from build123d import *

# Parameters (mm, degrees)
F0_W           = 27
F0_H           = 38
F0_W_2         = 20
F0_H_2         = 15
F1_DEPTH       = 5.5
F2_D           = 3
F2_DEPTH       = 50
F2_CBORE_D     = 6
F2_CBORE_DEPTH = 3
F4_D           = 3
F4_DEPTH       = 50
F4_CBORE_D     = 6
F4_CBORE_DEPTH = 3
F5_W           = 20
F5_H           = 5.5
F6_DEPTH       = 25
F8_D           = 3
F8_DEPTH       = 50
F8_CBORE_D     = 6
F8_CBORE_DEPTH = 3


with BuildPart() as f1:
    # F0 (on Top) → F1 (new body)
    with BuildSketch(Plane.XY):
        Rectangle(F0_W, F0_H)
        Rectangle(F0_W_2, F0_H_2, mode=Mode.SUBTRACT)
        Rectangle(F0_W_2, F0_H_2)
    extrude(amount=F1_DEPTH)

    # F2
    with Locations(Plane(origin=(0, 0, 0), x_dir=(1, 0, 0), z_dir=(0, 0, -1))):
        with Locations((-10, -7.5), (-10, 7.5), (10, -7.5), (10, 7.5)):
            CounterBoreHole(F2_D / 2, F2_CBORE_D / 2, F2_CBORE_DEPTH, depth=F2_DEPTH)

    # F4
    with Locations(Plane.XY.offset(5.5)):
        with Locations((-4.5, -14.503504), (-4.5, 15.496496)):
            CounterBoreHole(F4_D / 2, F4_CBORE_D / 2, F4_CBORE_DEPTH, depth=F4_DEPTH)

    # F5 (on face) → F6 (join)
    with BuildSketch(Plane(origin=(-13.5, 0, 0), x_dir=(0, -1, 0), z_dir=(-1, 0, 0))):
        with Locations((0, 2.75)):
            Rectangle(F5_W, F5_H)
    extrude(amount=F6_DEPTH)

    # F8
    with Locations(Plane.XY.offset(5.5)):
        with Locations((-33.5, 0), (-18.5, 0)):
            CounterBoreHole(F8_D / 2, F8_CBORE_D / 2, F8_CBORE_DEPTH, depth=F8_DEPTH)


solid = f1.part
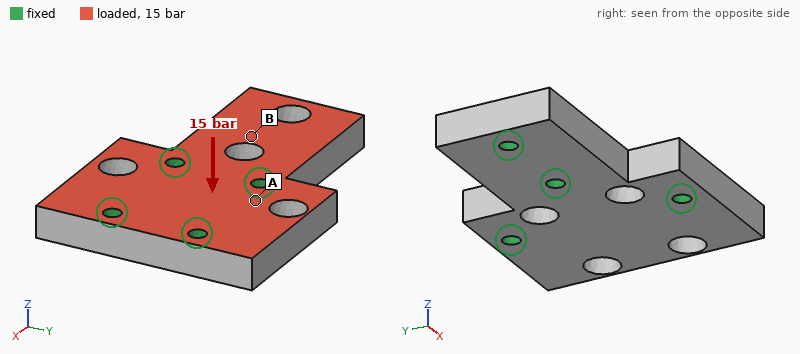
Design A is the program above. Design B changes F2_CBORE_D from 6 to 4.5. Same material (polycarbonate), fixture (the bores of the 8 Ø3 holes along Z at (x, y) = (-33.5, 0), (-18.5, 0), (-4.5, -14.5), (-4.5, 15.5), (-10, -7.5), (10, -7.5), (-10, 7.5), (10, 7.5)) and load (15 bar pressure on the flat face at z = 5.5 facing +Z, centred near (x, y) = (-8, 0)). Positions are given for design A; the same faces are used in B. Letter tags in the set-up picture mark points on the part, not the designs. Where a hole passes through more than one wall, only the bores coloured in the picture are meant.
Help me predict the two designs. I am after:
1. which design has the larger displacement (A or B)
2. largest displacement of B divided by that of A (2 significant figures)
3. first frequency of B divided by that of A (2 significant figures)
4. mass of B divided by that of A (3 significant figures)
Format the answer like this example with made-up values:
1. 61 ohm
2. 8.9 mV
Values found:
1. A
2. 0.88
3. 1.0
4. 1.02
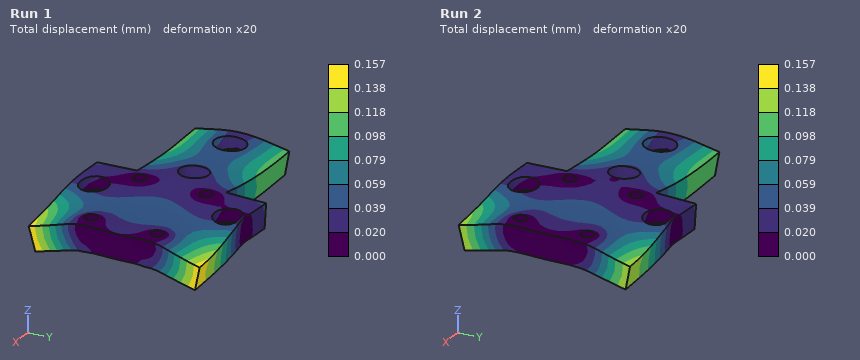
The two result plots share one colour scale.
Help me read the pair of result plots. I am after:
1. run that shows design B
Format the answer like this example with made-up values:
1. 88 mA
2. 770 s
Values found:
1. Run 2
